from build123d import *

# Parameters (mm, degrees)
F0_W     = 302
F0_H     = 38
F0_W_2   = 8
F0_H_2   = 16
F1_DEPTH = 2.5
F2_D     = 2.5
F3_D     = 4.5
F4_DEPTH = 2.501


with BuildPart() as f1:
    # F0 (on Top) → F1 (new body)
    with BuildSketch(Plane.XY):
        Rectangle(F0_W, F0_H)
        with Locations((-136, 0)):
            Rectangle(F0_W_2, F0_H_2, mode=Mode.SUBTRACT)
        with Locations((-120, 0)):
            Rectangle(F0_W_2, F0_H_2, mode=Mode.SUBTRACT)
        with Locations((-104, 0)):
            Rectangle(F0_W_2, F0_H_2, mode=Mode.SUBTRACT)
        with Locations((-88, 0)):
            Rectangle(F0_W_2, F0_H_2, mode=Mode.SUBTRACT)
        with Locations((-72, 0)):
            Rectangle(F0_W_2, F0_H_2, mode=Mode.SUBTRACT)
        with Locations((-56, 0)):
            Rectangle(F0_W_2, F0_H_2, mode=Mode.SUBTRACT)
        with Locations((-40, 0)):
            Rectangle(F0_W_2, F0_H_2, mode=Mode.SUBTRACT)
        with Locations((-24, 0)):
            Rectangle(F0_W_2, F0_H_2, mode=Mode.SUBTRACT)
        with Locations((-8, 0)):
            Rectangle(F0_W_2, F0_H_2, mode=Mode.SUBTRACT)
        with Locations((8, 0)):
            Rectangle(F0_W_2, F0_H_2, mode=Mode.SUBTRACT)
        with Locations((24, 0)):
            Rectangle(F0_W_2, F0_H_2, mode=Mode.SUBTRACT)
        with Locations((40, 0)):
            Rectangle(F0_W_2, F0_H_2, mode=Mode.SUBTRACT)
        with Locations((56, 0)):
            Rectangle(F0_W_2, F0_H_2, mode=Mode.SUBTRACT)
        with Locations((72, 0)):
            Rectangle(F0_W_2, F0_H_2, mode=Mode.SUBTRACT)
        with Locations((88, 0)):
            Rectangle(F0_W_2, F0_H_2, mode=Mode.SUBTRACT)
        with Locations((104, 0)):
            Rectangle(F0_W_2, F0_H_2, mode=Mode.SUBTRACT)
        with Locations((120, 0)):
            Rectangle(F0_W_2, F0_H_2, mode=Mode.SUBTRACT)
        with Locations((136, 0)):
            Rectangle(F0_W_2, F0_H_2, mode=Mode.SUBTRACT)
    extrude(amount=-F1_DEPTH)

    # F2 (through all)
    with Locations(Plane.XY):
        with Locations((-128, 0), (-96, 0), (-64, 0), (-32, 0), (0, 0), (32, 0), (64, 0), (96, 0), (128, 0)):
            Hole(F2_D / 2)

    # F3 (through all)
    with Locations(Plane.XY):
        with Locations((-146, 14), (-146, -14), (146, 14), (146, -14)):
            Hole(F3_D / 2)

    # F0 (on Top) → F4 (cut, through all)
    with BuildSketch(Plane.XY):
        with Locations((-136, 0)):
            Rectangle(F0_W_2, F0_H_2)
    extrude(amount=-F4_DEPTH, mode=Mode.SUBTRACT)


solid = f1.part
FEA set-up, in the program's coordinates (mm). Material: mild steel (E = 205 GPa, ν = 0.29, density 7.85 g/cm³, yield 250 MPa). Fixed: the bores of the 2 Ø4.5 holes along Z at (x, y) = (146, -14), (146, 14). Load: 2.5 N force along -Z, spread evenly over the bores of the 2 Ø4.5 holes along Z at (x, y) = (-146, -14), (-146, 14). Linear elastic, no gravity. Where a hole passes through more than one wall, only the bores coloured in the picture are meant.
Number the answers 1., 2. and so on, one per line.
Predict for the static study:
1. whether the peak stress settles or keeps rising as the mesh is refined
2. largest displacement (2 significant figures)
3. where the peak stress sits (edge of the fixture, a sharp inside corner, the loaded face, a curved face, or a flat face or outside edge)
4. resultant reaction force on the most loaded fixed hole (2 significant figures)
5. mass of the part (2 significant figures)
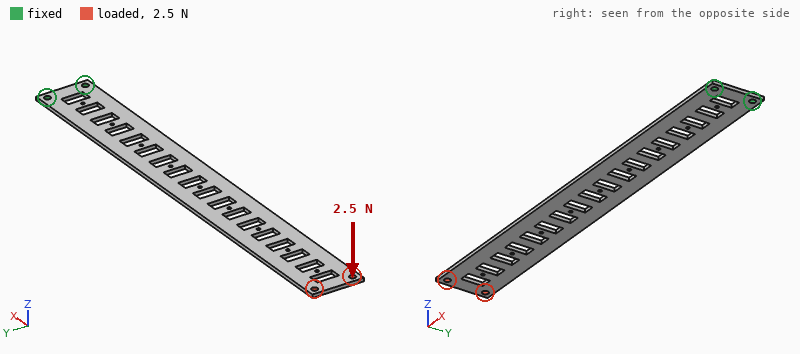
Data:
1. keeps rising
2. 3.4 mm
3. edge of the fixture
4. 1.3 N
5. 180 g
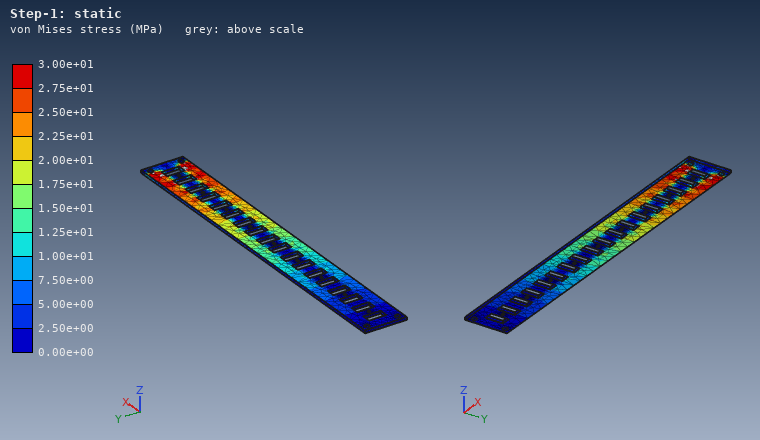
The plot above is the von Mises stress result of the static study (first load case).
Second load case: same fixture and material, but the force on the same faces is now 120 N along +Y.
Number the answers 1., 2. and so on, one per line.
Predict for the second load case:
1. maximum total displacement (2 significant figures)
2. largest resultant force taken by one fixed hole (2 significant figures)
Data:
1. 0.50 mm
2. 1.2 kN
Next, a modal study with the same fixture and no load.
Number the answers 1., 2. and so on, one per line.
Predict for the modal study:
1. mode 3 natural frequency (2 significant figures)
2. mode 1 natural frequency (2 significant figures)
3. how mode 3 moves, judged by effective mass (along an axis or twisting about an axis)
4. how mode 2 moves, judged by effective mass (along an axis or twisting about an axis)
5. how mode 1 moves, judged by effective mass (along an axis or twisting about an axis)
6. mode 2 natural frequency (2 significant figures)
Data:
1. 310 Hz
2. 21 Hz
3. twisting about X
4. along Z
5. along Z
6. 130 Hz
